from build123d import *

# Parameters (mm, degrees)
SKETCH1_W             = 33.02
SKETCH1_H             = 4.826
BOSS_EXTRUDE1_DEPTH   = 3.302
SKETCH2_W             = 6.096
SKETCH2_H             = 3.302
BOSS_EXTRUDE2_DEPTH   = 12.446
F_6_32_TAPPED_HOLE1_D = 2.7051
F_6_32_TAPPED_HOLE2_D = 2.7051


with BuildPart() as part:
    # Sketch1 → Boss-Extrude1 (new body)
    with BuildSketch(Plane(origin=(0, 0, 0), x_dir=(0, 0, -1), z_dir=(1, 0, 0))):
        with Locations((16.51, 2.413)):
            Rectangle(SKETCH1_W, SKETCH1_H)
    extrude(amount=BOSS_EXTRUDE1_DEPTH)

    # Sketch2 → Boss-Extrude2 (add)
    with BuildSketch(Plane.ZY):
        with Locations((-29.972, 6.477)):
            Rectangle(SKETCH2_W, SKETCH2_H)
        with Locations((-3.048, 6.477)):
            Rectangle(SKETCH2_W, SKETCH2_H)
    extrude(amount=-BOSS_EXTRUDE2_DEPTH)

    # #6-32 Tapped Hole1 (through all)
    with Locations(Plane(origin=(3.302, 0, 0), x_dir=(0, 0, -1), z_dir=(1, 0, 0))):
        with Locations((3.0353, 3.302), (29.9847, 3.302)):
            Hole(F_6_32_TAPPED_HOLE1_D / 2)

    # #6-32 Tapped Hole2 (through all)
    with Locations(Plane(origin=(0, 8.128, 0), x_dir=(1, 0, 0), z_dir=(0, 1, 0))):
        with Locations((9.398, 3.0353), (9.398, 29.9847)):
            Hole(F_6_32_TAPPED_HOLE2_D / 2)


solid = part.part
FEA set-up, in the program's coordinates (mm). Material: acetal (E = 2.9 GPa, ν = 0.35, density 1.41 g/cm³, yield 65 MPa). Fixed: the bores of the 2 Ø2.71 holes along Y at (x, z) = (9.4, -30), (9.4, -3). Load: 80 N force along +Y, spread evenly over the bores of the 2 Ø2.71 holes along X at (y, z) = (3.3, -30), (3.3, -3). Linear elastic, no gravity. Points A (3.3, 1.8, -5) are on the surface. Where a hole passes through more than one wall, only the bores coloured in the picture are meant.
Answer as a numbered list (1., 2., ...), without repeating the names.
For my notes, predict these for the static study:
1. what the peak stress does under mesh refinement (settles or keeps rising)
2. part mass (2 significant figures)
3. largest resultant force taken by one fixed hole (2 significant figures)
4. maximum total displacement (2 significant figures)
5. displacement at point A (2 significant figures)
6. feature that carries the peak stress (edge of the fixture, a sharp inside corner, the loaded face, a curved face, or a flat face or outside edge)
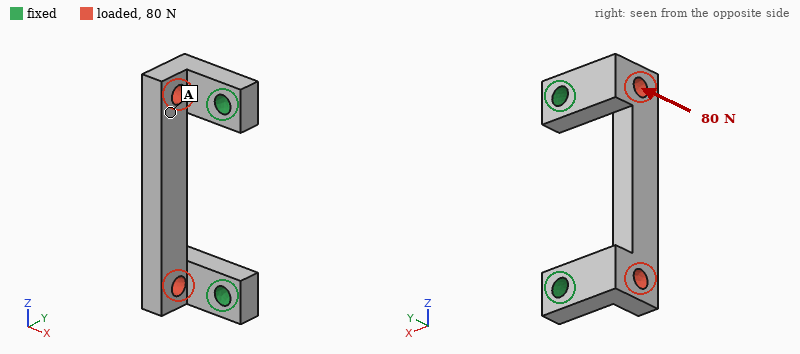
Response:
1. keeps rising
2. 1.3 g
3. 40 N
4. 0.18 mm
5. 0.11 mm
6. edge of the fixture
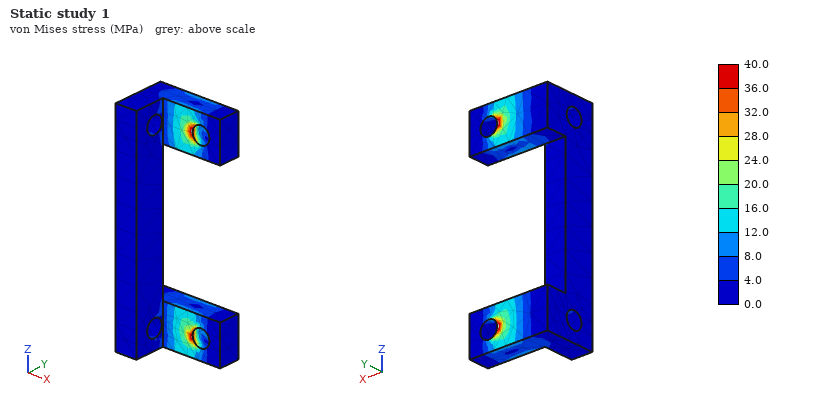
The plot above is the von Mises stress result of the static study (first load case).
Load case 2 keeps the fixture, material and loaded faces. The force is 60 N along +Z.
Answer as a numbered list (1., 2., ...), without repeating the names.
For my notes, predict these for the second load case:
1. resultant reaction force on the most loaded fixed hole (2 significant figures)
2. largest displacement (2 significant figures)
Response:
1. 31 N
2. 64 µm
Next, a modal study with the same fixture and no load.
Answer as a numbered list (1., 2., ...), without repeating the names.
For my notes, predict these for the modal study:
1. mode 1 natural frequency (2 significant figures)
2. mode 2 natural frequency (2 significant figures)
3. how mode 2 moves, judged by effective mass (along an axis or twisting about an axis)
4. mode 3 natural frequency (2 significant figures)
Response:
1. 3200 Hz
2. 5300 Hz
3. along Z
4. 5900 Hz
